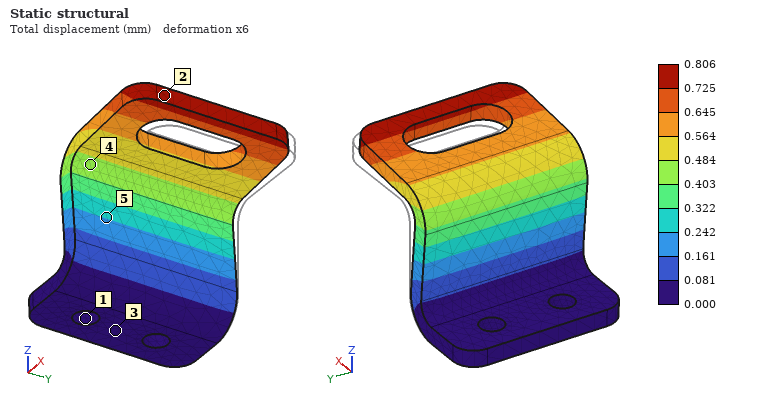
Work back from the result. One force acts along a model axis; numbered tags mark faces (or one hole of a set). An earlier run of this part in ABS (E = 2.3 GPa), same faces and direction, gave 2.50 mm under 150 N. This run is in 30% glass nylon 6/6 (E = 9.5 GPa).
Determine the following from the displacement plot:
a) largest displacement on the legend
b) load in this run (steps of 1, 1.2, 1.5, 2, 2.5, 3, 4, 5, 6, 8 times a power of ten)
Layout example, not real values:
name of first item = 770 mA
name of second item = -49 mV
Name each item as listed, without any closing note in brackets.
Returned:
largest displacement on the legend = 0.806 mm
load in this run = 200 N
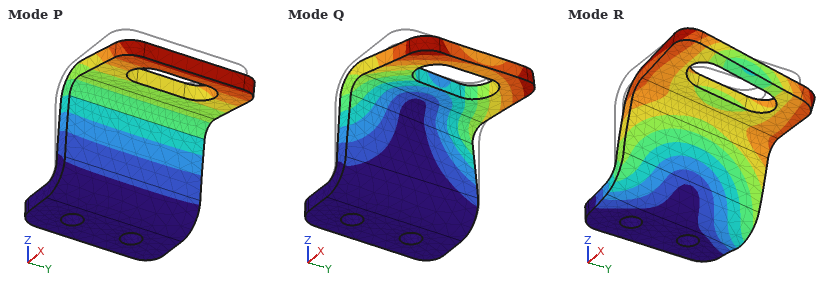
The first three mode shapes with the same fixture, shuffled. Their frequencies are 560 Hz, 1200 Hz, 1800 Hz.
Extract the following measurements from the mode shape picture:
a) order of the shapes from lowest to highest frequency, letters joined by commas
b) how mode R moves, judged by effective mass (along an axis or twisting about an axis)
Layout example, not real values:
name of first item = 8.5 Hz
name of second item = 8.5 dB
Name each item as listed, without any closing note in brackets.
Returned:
order of the shapes from lowest to highest frequency, letters joined by commas = P, Q, R
how mode R moves, judged by effective mass = along Y
